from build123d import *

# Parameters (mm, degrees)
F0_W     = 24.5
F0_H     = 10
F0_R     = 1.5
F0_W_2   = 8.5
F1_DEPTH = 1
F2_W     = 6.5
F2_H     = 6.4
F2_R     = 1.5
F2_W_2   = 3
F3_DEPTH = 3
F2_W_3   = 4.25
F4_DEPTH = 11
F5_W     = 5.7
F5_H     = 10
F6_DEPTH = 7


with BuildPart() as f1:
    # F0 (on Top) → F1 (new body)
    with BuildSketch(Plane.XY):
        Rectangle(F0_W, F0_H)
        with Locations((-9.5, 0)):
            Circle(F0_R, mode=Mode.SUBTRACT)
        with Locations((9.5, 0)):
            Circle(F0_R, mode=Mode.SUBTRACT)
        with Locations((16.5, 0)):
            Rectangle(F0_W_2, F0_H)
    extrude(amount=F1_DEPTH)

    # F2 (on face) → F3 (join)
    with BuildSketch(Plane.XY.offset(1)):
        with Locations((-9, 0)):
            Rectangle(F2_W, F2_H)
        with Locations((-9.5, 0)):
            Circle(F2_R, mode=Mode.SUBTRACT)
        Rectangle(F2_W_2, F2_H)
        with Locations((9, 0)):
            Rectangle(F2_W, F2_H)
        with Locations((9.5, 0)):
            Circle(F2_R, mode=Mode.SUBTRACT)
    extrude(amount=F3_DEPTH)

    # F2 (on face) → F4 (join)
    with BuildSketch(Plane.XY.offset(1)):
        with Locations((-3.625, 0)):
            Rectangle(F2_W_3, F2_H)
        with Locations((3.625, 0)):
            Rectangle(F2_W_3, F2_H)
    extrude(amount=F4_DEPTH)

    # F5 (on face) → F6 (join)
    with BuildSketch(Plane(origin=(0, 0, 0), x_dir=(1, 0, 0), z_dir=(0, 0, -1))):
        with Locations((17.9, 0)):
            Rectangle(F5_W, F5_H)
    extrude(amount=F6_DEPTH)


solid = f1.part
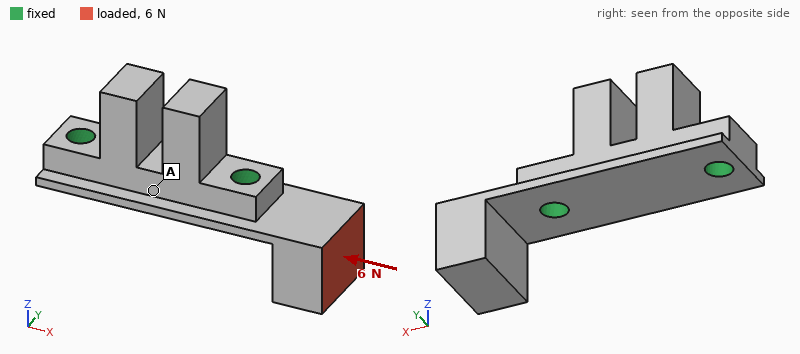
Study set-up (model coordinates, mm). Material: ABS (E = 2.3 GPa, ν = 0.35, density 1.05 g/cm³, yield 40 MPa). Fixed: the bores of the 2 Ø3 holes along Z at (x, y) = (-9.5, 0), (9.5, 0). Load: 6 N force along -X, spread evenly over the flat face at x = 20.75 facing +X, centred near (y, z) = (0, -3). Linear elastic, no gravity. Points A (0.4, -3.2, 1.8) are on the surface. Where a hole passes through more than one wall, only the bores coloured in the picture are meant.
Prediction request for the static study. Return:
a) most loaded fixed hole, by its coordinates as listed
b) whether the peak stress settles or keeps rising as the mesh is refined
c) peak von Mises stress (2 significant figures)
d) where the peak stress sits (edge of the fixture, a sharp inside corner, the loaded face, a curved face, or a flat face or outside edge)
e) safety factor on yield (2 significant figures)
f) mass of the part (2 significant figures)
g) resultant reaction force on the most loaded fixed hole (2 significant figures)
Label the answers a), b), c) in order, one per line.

a) (9.5, 0)
b) settles
c) 14 MPa
d) a flat face or outside edge
e) 2.9
f) 1.7 g
g) 5.5 N
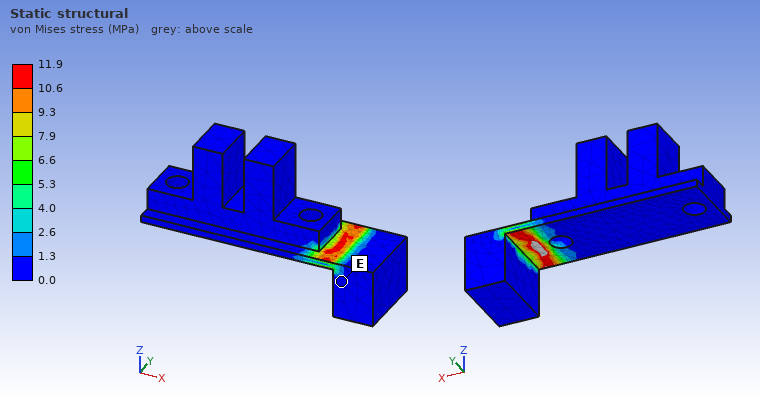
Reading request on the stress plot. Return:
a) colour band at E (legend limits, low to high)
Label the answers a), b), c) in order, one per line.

a) 0.0 to 1.3 MPa
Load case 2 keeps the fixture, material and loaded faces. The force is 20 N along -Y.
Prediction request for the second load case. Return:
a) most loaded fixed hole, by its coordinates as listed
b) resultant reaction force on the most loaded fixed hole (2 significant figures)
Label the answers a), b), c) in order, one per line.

a) (9.5, 0)
b) 25 N
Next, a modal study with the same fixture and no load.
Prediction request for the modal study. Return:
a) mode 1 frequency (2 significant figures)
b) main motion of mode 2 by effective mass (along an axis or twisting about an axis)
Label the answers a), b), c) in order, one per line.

a) 830 Hz
b) along Y
